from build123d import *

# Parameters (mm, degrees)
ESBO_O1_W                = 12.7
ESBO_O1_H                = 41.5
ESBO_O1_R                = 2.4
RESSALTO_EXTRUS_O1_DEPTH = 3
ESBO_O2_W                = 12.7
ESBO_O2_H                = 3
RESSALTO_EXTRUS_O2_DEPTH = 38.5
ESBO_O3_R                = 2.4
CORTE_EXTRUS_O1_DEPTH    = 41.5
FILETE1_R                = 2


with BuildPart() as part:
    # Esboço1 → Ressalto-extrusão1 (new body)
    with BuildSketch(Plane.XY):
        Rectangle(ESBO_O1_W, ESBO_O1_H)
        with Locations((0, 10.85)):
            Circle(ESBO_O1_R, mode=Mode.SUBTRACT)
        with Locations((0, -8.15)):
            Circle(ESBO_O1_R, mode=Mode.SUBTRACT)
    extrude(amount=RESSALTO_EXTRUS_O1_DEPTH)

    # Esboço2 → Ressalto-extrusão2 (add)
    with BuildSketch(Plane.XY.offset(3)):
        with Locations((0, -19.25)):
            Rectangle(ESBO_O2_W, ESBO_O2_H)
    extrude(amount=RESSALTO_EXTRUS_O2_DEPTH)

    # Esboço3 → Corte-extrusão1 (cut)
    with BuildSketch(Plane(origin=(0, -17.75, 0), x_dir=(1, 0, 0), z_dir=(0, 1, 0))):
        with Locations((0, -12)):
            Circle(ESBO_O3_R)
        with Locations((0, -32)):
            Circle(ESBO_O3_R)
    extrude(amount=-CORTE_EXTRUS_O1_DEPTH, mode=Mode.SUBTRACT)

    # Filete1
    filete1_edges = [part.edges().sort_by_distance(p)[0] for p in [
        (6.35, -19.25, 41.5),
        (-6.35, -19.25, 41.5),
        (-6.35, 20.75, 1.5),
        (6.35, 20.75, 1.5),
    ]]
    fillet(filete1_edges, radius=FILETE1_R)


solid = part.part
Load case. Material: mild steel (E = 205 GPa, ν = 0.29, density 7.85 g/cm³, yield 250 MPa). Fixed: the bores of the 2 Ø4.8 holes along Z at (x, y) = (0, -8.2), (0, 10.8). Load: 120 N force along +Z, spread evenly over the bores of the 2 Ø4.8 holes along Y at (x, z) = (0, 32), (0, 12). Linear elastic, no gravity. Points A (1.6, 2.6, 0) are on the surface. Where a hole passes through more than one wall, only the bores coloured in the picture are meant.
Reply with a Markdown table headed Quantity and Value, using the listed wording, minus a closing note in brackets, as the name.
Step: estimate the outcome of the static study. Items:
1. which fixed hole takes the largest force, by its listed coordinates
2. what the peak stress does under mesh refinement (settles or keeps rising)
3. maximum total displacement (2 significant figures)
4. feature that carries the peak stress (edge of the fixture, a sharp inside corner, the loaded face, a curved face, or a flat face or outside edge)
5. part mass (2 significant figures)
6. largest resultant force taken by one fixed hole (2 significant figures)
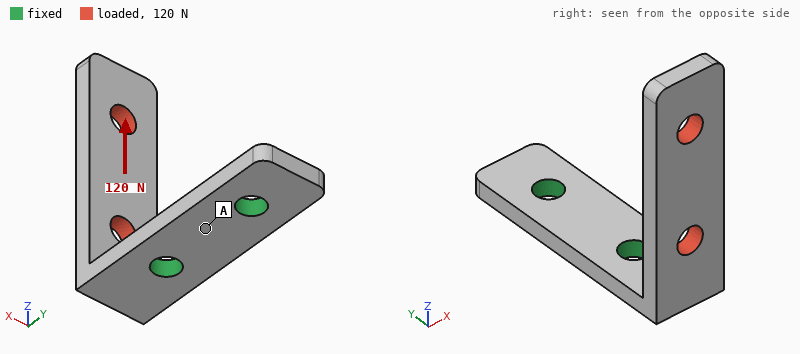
| Quantity | Value |
|---|---|
| which fixed hole takes the largest force, by its listed coordinates | (0, -8.2) |
| what the peak stress does under mesh refinement | keeps rising |
| maximum total displacement | 39 µm |
| feature that carries the peak stress | edge of the fixture |
| part mass | 22 g |
| largest resultant force taken by one fixed hole | 120 N |
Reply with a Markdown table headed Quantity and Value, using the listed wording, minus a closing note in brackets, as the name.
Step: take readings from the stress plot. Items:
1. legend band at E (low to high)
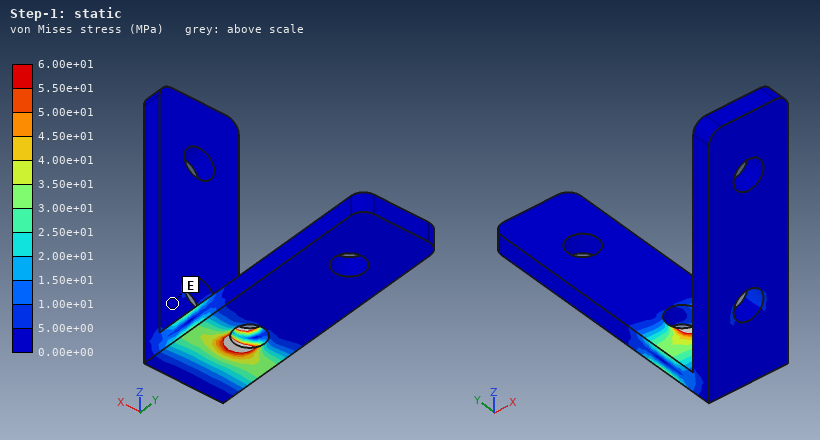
| Quantity | Value |
|---|---|
| legend band at E | 0.00e+00 to 5.00e+00 MPa |
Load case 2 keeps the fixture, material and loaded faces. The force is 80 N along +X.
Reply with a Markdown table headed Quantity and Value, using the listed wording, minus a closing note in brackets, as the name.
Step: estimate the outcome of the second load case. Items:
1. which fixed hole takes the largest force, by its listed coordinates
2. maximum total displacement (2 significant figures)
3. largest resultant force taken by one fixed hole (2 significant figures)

| Quantity | Value |
|---|---|
| which fixed hole takes the largest force, by its listed coordinates | (0, -8.2) |
| maximum total displacement | 67 µm |
| largest resultant force taken by one fixed hole | 96 N |
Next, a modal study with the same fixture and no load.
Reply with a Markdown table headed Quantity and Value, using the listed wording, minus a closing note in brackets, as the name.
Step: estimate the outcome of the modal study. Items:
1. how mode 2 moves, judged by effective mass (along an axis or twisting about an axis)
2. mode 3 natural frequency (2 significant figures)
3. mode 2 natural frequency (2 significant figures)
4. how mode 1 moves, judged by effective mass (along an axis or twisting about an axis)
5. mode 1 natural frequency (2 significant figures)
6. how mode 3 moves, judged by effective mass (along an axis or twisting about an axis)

| Quantity | Value |
|---|---|
| how mode 2 moves, judged by effective mass | along X |
| mode 3 natural frequency | 6300 Hz |
| mode 2 natural frequency | 2000 Hz |
| how mode 1 moves, judged by effective mass | along Y |
| mode 1 natural frequency | 1100 Hz |
| how mode 3 moves, judged by effective mass | along Z |
